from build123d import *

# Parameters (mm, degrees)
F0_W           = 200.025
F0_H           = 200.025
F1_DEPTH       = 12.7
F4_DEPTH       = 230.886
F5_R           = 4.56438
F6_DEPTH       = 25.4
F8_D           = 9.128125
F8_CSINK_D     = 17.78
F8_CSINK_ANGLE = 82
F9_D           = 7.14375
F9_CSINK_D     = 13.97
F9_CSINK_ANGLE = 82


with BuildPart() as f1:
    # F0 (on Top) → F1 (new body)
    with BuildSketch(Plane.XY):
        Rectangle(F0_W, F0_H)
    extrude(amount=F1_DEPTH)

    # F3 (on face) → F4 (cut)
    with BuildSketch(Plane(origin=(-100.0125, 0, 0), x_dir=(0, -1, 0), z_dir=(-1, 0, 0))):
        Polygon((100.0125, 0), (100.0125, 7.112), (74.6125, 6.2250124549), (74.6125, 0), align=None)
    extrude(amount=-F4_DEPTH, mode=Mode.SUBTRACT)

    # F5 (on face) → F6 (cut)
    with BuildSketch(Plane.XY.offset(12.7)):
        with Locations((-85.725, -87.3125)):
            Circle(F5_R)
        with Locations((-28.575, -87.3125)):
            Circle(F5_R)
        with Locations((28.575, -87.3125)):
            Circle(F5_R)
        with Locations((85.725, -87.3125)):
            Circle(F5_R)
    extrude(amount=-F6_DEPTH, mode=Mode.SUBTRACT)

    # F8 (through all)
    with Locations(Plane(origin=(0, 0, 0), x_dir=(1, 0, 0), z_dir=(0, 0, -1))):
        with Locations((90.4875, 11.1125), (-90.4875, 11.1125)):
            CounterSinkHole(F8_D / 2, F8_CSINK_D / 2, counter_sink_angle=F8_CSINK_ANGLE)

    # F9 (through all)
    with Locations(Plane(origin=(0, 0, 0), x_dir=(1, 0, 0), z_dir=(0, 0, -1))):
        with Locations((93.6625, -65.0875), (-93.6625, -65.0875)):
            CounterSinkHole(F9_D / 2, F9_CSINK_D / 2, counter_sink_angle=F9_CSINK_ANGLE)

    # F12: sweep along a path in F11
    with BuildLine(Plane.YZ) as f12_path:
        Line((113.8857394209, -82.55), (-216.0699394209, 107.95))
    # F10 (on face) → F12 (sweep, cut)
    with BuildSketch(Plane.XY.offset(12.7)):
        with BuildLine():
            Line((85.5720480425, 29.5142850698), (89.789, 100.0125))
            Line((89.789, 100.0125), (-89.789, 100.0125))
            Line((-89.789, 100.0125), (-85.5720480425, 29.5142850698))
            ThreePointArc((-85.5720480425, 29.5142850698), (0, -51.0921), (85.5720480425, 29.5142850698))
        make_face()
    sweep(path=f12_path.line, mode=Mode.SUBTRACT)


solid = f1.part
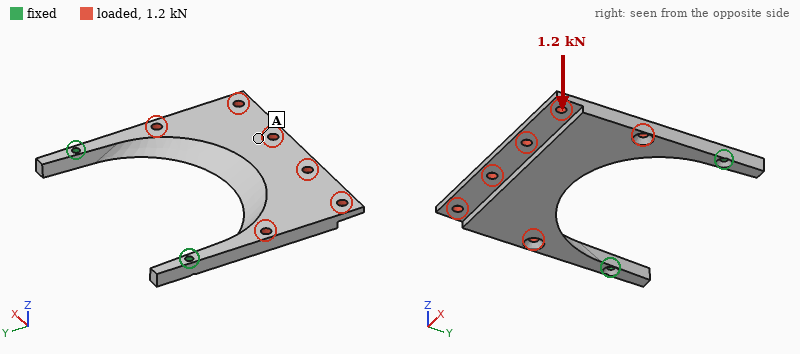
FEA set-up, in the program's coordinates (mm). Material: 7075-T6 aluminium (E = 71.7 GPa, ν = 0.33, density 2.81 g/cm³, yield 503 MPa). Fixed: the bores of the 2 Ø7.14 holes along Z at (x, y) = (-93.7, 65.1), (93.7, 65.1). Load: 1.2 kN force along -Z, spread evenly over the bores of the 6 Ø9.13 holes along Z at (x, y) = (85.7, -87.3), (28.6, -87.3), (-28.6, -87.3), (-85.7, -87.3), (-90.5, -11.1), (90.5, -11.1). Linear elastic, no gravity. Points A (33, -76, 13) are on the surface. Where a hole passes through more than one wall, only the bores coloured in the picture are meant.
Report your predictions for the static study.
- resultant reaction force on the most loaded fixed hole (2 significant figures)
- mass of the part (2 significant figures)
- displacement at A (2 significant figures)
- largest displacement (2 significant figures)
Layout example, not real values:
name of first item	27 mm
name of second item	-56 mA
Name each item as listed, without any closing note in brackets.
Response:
resultant reaction force on the most loaded fixed hole	600 N
mass of the part	570 g
displacement at A	2.6 mm
largest displacement	3.2 mm
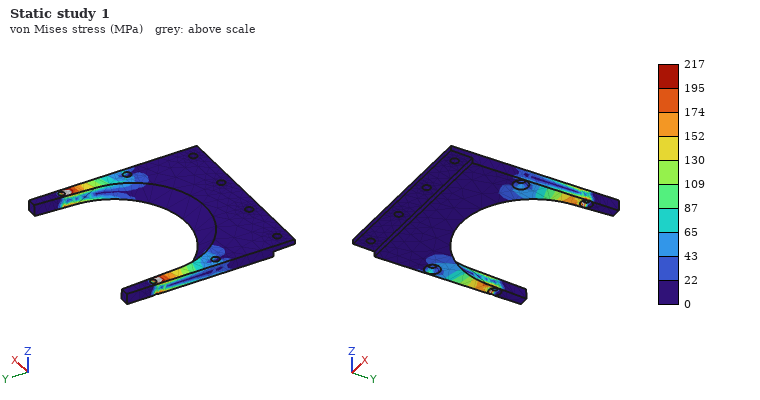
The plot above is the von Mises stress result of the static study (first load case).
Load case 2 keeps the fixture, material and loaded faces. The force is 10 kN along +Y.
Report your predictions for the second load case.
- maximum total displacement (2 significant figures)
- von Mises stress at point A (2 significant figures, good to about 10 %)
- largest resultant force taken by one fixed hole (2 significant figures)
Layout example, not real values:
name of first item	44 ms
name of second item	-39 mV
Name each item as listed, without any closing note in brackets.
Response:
maximum total displacement	0.89 mm
von Mises stress at point A	9.7 MPa
largest resultant force taken by one fixed hole	5.0 kN
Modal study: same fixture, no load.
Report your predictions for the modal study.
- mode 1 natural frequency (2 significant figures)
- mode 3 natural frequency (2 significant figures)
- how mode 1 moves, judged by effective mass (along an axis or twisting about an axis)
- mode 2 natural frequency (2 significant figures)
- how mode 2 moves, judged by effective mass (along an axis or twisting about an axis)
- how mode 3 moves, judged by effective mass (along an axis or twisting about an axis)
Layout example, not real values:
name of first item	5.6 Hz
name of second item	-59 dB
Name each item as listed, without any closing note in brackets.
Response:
mode 1 natural frequency	180 Hz
mode 3 natural frequency	990 Hz
how mode 1 moves, judged by effective mass	along Z
mode 2 natural frequency	530 Hz
how mode 2 moves, judged by effective mass	twisting about Y
how mode 3 moves, judged by effective mass	along X
